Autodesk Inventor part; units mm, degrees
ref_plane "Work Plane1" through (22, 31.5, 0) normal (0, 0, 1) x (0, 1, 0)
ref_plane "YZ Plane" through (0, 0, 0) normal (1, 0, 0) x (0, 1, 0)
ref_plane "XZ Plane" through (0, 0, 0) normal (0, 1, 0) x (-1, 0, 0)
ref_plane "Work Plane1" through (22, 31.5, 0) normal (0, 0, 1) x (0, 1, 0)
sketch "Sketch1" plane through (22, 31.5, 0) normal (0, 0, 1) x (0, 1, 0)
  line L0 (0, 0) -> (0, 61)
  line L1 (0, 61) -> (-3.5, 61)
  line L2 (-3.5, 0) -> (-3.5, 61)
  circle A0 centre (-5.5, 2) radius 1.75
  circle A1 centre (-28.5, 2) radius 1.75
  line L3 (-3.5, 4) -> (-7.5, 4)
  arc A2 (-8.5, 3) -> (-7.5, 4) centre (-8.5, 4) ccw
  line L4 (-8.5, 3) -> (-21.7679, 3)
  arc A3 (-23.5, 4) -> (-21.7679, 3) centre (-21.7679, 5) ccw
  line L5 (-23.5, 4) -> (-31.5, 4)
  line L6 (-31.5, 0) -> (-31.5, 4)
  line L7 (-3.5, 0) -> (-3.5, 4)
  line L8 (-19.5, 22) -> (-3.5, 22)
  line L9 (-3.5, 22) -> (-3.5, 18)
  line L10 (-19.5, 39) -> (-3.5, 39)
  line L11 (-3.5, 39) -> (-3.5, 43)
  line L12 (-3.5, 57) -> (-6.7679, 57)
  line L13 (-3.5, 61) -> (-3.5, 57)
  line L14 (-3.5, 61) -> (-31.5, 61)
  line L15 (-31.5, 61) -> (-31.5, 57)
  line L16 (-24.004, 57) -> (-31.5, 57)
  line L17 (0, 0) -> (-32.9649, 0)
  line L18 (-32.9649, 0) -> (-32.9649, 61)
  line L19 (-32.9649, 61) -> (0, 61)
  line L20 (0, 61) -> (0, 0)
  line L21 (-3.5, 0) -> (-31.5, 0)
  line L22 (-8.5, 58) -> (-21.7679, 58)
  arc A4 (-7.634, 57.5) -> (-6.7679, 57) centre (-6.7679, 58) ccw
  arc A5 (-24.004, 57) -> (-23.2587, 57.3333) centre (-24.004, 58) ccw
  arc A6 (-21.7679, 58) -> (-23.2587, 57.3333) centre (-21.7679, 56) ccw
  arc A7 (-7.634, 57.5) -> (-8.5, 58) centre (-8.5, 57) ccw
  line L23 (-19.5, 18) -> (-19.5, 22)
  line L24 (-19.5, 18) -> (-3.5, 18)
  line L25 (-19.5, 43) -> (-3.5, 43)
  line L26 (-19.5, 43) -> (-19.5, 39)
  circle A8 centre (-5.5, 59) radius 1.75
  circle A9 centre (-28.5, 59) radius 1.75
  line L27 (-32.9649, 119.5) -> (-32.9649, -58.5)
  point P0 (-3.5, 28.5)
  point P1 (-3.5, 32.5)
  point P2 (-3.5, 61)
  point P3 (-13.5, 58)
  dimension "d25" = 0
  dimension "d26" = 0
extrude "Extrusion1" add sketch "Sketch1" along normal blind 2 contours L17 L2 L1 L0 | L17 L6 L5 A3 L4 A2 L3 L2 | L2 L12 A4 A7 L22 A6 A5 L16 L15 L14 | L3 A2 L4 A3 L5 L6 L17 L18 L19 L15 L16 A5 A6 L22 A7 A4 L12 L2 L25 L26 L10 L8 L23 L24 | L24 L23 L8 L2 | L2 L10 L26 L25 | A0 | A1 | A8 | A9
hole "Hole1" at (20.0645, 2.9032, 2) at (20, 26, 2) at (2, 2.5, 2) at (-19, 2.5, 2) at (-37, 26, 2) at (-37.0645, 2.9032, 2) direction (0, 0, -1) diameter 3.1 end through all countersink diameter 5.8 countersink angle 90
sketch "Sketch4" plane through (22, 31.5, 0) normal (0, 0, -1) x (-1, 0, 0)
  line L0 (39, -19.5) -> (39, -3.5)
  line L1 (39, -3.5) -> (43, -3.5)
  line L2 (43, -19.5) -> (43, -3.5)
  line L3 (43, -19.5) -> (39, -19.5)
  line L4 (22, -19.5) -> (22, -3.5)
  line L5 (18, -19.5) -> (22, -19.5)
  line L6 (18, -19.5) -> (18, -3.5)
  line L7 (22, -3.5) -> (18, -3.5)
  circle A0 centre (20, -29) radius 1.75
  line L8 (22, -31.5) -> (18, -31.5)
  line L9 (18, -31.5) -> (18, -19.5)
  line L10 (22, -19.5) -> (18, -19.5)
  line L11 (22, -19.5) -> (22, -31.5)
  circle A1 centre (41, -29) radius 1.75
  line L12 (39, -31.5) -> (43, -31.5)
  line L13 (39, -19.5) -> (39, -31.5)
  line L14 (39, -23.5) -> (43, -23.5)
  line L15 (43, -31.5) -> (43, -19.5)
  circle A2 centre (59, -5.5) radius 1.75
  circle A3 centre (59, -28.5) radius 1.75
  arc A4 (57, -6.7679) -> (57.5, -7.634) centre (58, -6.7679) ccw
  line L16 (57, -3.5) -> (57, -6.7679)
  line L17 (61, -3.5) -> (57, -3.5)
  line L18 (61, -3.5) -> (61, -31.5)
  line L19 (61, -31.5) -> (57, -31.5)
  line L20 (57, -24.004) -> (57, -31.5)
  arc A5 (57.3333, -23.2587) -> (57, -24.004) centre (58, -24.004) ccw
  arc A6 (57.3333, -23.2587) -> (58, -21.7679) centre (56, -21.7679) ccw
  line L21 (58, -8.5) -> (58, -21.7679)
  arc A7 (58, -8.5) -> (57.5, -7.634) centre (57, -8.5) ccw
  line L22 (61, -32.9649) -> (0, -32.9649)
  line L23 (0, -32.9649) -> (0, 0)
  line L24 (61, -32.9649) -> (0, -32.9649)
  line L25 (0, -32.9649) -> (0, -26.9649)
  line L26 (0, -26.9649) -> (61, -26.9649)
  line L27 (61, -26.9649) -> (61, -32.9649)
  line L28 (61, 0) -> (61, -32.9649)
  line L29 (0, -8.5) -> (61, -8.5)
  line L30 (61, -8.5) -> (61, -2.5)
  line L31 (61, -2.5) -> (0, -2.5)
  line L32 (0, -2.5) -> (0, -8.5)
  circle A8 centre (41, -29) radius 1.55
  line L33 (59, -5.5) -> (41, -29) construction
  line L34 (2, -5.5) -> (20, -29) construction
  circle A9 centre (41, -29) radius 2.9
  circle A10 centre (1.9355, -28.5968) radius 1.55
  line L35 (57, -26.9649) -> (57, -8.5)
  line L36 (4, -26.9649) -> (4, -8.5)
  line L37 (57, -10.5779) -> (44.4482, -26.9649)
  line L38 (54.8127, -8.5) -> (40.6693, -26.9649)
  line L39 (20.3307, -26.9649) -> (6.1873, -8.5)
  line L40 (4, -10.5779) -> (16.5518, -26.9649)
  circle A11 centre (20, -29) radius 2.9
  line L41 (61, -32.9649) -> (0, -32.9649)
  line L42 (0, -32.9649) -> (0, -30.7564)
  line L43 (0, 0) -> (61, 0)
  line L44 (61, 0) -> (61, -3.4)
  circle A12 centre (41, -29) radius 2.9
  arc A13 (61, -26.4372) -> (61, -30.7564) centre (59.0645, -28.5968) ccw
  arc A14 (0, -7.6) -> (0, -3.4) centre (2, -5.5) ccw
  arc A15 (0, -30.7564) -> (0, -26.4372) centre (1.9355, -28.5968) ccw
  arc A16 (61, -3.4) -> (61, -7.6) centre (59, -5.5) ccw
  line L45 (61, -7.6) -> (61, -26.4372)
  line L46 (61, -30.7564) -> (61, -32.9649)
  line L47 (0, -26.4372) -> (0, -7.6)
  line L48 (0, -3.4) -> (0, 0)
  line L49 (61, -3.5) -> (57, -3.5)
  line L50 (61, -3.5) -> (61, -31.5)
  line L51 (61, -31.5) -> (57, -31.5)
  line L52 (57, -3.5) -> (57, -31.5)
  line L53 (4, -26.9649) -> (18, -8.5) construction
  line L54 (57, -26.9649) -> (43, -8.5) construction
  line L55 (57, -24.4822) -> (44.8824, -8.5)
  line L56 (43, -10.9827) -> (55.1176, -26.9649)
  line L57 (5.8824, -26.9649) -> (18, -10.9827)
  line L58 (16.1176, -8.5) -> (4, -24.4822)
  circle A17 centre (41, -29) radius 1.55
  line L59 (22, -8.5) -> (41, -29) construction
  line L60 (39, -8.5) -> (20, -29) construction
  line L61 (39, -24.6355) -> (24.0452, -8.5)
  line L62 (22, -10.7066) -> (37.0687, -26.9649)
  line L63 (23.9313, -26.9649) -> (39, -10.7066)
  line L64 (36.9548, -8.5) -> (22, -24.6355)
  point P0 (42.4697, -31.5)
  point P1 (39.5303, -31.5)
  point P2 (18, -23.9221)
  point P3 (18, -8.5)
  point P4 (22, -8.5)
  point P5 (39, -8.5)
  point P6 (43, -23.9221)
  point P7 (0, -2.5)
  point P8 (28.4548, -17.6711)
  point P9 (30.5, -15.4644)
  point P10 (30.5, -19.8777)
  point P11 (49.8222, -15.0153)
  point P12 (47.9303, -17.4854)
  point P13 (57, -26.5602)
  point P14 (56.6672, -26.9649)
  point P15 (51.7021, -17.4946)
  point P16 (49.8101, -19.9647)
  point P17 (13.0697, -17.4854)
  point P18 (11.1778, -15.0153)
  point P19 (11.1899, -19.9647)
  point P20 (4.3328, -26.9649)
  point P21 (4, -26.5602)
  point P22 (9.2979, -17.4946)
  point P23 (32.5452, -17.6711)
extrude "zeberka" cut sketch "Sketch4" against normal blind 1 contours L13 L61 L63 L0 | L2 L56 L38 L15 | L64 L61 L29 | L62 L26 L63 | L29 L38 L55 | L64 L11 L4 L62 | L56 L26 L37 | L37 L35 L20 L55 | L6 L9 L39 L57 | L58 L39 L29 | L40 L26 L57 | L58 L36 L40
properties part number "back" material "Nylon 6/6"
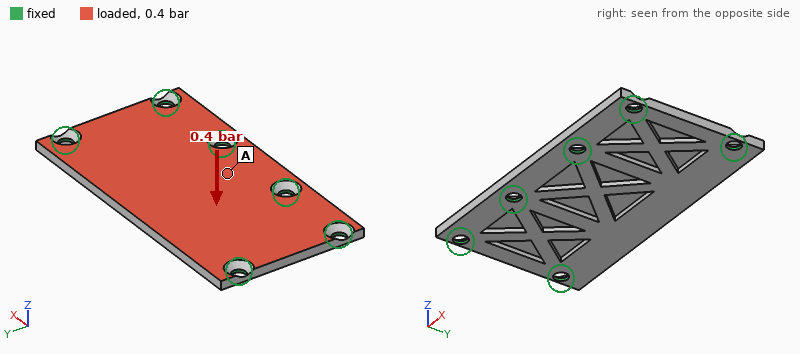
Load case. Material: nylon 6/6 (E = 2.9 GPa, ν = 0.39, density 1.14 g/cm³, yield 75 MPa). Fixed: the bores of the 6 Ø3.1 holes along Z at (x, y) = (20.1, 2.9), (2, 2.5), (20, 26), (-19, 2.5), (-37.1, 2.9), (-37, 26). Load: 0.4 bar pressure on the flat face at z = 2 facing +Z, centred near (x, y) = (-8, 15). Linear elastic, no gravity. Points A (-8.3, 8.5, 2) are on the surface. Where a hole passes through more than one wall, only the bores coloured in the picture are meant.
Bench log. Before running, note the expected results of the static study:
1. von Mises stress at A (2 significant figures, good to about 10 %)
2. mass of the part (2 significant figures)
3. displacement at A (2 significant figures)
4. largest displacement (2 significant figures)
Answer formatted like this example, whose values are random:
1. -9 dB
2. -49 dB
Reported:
1. 3.3 MPa
2. 3.9 g
3. 0.13 mm
4. 0.66 mm
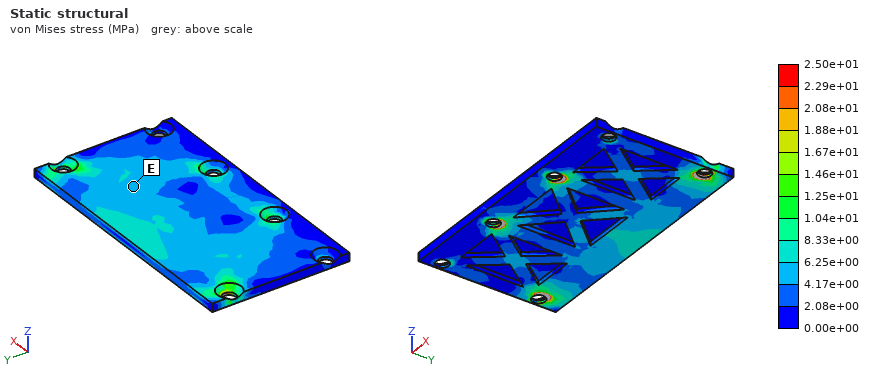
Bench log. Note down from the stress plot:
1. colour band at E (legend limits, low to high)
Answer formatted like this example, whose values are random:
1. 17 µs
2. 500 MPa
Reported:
1. 4.17e+00 to 6.25e+00 MPa
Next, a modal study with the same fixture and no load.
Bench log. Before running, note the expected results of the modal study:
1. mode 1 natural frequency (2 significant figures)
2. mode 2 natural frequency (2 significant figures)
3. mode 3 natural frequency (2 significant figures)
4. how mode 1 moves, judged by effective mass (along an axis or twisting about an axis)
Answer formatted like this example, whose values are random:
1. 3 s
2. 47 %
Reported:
1. 1100 Hz
2. 2600 Hz
3. 3400 Hz
4. along Z
